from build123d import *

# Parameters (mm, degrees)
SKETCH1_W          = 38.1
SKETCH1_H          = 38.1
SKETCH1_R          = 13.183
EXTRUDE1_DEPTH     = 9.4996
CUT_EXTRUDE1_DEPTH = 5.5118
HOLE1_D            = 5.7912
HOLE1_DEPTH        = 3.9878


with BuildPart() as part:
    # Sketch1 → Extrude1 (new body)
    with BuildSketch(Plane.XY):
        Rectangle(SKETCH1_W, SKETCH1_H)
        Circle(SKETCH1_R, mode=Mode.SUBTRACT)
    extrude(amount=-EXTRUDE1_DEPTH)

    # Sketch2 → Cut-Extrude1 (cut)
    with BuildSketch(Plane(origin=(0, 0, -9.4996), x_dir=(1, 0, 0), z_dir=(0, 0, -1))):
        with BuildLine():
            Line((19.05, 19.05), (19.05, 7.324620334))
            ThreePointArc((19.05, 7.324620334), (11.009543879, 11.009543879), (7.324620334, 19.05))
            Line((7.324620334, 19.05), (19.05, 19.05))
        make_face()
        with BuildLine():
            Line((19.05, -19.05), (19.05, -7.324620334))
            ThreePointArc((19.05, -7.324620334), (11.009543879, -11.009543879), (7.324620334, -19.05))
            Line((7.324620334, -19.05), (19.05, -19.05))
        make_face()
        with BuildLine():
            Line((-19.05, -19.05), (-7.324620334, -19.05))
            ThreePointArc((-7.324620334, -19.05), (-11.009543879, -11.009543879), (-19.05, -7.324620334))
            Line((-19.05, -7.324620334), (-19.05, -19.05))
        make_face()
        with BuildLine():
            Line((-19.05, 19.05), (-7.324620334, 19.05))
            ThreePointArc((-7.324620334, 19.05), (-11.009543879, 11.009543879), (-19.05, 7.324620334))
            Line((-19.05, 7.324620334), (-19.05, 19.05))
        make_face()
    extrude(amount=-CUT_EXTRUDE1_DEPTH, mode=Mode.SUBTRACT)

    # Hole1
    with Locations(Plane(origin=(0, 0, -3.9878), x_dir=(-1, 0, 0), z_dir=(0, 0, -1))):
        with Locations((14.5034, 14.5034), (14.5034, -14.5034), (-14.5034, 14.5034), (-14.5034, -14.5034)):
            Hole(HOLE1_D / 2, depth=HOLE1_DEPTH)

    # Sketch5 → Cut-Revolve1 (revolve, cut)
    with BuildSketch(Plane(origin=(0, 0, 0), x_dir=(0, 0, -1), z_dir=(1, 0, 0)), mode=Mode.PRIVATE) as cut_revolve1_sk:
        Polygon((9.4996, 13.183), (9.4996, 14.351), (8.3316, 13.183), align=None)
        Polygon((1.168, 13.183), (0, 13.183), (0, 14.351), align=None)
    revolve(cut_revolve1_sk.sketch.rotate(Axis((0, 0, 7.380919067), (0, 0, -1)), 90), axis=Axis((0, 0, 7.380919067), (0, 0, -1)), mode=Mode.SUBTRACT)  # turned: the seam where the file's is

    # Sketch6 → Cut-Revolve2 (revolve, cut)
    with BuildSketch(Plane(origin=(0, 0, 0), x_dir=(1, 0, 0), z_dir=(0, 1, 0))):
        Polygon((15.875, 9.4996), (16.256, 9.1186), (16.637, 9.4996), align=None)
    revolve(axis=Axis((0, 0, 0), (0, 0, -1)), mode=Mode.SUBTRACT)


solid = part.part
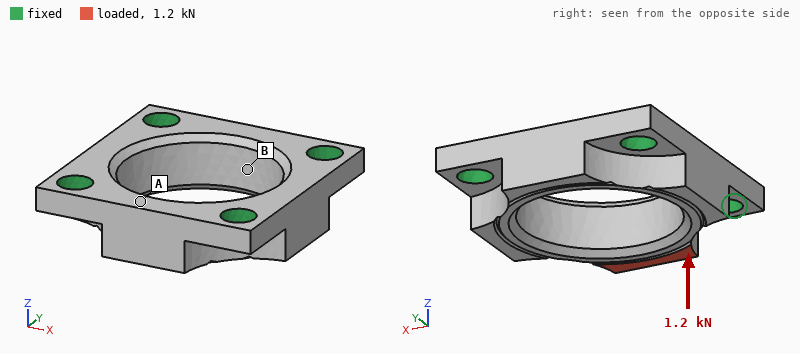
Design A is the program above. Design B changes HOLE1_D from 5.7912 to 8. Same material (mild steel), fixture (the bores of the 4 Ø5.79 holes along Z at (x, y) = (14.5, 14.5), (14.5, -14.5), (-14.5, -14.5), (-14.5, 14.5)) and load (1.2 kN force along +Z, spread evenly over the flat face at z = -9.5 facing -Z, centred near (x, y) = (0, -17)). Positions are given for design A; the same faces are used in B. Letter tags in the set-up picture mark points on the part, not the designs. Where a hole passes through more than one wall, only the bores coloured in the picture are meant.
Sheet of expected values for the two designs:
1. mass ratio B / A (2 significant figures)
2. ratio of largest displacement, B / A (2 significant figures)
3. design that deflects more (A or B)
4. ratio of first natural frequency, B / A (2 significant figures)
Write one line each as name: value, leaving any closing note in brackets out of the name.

mass ratio B / A: 0.93
ratio of largest displacement, B / A: 0.78
design that deflects more: A
ratio of first natural frequency, B / A: 1.2
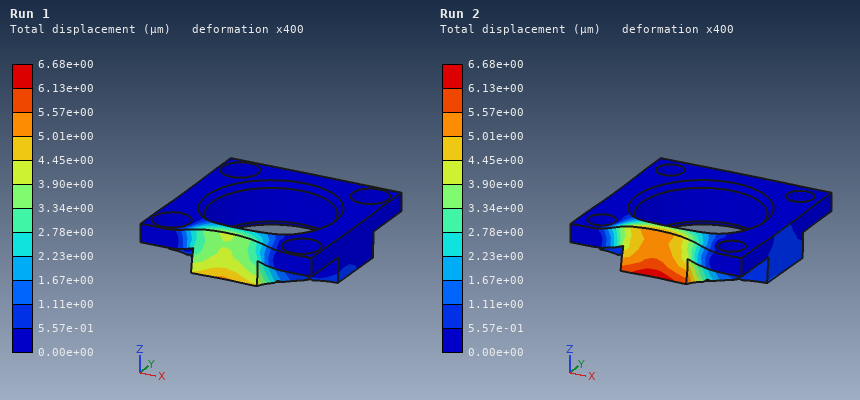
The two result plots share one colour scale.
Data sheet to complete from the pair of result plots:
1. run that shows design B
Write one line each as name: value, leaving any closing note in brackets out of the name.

run that shows design B: Run 1
